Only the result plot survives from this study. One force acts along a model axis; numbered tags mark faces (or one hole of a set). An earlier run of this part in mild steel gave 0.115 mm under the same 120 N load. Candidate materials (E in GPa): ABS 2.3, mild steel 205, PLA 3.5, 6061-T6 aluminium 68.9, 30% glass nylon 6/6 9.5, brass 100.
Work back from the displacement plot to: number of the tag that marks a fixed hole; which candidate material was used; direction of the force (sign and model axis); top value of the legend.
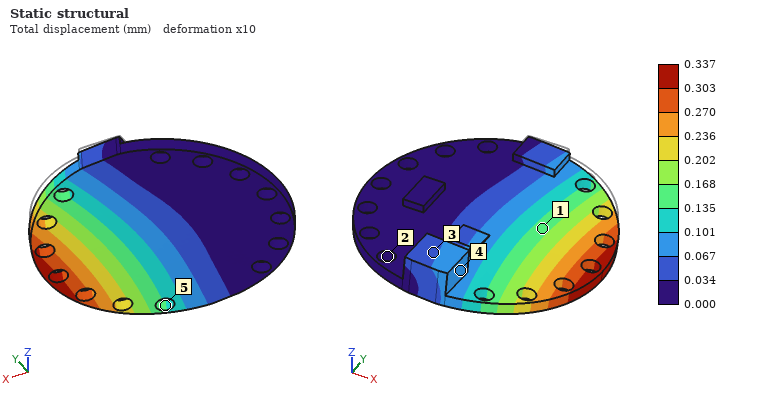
2
6061-T6 aluminium
-Z
0.337 mm
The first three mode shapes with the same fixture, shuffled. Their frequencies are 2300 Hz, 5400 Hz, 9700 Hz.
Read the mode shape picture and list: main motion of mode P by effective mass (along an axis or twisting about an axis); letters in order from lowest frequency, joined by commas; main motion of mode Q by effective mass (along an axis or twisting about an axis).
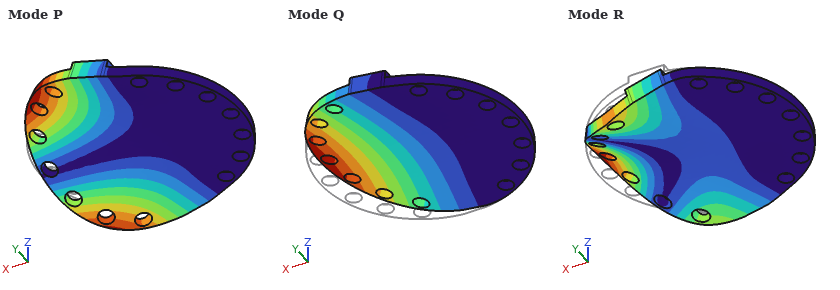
twisting about X
Q, P, R
along Z
